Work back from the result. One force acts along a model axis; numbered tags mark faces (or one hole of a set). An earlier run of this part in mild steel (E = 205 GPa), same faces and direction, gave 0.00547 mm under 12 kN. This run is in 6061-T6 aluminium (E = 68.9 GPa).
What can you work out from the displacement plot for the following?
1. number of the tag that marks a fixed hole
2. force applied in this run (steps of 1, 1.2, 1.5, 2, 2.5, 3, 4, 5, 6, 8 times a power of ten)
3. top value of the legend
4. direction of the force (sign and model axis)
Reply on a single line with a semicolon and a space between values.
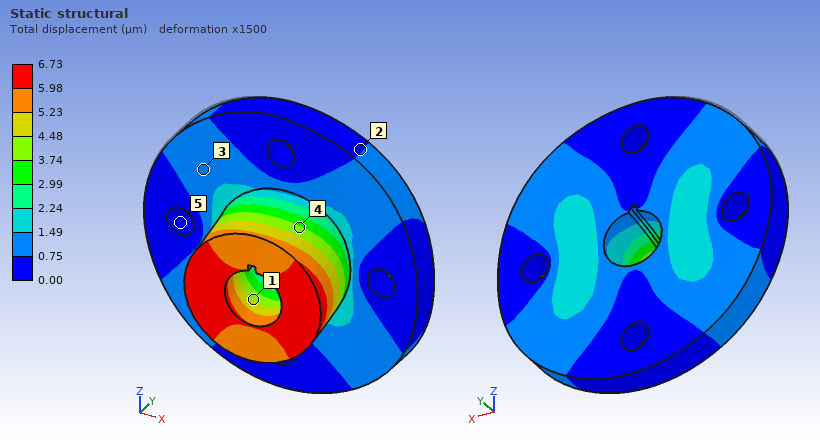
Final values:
5; 5 kN; 6.73 µm; +X
